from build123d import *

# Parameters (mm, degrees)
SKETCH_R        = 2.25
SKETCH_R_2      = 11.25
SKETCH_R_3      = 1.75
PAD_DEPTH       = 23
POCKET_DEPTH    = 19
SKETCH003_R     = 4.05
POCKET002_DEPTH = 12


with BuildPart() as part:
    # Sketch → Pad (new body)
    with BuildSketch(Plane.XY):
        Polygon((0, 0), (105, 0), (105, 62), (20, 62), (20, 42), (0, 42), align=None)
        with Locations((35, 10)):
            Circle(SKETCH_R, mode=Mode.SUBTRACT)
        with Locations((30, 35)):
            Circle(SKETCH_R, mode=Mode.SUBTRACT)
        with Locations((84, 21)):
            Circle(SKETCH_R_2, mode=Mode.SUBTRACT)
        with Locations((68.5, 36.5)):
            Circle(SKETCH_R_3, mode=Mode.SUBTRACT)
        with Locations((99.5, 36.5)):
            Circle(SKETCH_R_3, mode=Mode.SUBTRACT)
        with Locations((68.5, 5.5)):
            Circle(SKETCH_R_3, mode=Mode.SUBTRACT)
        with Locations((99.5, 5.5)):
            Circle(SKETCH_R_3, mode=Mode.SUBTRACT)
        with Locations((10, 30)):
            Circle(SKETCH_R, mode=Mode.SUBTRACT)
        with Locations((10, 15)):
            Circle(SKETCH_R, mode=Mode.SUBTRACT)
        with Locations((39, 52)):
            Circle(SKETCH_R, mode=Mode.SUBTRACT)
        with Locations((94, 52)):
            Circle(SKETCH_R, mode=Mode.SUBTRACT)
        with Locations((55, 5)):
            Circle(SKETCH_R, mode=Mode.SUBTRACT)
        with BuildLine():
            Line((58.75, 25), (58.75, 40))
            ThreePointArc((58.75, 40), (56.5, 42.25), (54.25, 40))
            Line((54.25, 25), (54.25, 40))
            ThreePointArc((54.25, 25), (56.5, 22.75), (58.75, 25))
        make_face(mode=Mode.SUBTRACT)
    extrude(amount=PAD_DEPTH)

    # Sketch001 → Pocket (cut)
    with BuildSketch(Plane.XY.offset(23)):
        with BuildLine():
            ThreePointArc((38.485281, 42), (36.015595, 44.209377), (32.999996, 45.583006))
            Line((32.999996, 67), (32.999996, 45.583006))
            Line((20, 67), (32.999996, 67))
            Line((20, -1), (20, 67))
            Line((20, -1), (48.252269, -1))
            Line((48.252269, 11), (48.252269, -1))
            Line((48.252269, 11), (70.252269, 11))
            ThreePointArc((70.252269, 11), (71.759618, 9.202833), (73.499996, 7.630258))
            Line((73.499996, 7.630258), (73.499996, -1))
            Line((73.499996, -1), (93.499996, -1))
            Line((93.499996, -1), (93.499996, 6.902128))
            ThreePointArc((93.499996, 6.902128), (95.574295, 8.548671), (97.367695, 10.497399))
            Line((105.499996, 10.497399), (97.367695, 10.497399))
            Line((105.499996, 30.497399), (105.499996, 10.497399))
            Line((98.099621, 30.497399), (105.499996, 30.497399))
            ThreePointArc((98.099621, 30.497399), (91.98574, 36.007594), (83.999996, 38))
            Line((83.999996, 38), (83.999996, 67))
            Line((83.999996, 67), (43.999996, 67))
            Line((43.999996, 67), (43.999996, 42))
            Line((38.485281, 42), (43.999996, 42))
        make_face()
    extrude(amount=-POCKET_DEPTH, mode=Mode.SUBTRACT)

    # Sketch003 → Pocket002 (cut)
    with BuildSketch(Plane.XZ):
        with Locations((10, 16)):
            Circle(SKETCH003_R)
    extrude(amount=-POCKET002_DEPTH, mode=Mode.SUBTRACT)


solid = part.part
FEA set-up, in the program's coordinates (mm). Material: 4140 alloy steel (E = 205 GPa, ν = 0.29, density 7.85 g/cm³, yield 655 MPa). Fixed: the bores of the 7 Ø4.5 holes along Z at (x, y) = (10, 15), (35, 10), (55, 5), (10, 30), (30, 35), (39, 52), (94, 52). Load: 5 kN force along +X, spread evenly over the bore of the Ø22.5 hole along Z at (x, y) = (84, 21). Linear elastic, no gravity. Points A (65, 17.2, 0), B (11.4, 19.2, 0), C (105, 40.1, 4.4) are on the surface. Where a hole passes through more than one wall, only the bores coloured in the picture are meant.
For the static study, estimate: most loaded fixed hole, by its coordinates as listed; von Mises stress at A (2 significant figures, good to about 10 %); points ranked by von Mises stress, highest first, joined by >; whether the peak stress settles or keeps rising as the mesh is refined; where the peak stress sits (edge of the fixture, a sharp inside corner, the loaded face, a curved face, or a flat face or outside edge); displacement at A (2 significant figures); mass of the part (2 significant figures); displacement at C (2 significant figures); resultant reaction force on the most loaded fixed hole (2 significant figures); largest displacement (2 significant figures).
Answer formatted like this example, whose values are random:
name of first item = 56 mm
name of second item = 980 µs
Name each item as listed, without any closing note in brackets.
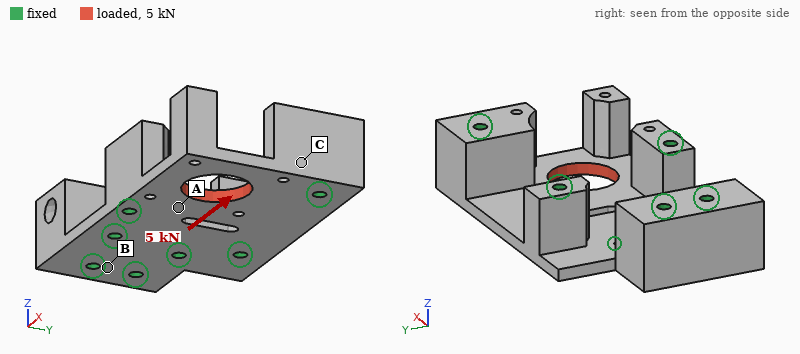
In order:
most loaded fixed hole, by its coordinates as listed = (55, 5)
von Mises stress at A = 24 MPa
points ranked by von Mises stress, highest first, joined by > = A > C > B
whether the peak stress settles or keeps rising as the mesh is refined = keeps rising
where the peak stress sits = a sharp inside corner
displacement at A = 2.3 µm
mass of the part = 450 g
displacement at C = 3.0 µm
resultant reaction force on the most loaded fixed hole = 2.2 kN
largest displacement = 8.8 µm
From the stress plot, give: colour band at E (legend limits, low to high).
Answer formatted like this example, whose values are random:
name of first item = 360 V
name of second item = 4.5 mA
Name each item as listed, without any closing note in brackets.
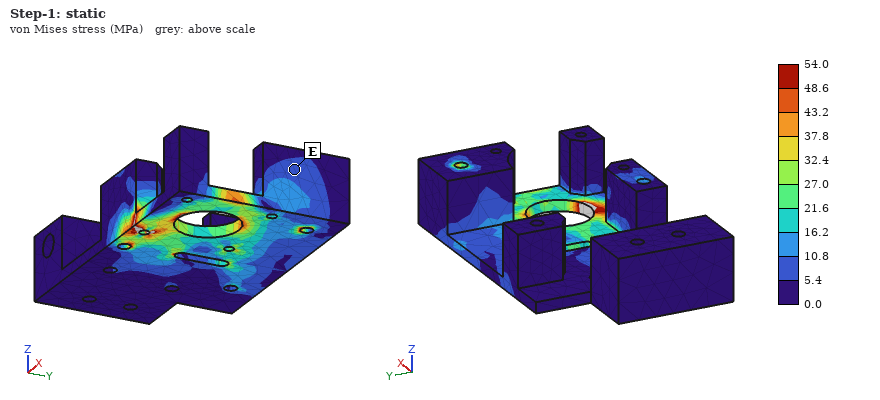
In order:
colour band at E = 5.4 to 10.8 MPa
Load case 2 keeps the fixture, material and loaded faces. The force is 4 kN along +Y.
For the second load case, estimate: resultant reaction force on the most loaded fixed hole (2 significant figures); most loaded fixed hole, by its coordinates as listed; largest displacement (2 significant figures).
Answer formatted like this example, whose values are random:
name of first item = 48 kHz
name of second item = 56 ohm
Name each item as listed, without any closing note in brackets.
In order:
resultant reaction force on the most loaded fixed hole = 2.5 kN
most loaded fixed hole, by its coordinates as listed = (94, 52)
largest displacement = 7.3 µm
